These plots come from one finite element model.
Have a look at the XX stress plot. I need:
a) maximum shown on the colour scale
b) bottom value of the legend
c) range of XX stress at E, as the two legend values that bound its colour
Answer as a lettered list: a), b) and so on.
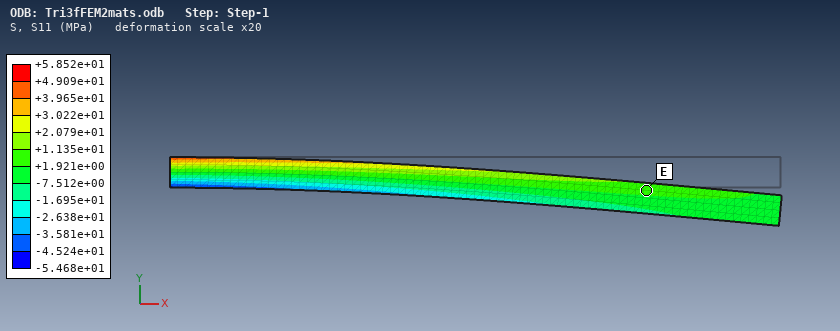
a) +5.852e+01 MPa
b) -5.468e+01 MPa
c) +1.921e+00 to +1.135e+01 MPa
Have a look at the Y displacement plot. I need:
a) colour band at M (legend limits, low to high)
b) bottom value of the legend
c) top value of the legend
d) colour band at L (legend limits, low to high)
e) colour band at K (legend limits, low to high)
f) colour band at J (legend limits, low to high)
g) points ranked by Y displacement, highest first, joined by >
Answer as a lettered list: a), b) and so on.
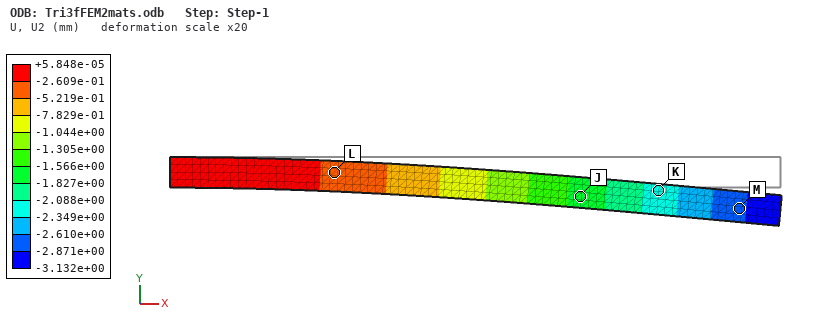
a) -2.871e+00 to -2.610e+00 mm
b) -3.132e+00 mm
c) +5.848e-05 mm
d) -5.219e-01 to -2.609e-01 mm
e) -2.349e+00 to -2.088e+00 mm
f) -1.827e+00 to -1.566e+00 mm
g) L > J > K > M
